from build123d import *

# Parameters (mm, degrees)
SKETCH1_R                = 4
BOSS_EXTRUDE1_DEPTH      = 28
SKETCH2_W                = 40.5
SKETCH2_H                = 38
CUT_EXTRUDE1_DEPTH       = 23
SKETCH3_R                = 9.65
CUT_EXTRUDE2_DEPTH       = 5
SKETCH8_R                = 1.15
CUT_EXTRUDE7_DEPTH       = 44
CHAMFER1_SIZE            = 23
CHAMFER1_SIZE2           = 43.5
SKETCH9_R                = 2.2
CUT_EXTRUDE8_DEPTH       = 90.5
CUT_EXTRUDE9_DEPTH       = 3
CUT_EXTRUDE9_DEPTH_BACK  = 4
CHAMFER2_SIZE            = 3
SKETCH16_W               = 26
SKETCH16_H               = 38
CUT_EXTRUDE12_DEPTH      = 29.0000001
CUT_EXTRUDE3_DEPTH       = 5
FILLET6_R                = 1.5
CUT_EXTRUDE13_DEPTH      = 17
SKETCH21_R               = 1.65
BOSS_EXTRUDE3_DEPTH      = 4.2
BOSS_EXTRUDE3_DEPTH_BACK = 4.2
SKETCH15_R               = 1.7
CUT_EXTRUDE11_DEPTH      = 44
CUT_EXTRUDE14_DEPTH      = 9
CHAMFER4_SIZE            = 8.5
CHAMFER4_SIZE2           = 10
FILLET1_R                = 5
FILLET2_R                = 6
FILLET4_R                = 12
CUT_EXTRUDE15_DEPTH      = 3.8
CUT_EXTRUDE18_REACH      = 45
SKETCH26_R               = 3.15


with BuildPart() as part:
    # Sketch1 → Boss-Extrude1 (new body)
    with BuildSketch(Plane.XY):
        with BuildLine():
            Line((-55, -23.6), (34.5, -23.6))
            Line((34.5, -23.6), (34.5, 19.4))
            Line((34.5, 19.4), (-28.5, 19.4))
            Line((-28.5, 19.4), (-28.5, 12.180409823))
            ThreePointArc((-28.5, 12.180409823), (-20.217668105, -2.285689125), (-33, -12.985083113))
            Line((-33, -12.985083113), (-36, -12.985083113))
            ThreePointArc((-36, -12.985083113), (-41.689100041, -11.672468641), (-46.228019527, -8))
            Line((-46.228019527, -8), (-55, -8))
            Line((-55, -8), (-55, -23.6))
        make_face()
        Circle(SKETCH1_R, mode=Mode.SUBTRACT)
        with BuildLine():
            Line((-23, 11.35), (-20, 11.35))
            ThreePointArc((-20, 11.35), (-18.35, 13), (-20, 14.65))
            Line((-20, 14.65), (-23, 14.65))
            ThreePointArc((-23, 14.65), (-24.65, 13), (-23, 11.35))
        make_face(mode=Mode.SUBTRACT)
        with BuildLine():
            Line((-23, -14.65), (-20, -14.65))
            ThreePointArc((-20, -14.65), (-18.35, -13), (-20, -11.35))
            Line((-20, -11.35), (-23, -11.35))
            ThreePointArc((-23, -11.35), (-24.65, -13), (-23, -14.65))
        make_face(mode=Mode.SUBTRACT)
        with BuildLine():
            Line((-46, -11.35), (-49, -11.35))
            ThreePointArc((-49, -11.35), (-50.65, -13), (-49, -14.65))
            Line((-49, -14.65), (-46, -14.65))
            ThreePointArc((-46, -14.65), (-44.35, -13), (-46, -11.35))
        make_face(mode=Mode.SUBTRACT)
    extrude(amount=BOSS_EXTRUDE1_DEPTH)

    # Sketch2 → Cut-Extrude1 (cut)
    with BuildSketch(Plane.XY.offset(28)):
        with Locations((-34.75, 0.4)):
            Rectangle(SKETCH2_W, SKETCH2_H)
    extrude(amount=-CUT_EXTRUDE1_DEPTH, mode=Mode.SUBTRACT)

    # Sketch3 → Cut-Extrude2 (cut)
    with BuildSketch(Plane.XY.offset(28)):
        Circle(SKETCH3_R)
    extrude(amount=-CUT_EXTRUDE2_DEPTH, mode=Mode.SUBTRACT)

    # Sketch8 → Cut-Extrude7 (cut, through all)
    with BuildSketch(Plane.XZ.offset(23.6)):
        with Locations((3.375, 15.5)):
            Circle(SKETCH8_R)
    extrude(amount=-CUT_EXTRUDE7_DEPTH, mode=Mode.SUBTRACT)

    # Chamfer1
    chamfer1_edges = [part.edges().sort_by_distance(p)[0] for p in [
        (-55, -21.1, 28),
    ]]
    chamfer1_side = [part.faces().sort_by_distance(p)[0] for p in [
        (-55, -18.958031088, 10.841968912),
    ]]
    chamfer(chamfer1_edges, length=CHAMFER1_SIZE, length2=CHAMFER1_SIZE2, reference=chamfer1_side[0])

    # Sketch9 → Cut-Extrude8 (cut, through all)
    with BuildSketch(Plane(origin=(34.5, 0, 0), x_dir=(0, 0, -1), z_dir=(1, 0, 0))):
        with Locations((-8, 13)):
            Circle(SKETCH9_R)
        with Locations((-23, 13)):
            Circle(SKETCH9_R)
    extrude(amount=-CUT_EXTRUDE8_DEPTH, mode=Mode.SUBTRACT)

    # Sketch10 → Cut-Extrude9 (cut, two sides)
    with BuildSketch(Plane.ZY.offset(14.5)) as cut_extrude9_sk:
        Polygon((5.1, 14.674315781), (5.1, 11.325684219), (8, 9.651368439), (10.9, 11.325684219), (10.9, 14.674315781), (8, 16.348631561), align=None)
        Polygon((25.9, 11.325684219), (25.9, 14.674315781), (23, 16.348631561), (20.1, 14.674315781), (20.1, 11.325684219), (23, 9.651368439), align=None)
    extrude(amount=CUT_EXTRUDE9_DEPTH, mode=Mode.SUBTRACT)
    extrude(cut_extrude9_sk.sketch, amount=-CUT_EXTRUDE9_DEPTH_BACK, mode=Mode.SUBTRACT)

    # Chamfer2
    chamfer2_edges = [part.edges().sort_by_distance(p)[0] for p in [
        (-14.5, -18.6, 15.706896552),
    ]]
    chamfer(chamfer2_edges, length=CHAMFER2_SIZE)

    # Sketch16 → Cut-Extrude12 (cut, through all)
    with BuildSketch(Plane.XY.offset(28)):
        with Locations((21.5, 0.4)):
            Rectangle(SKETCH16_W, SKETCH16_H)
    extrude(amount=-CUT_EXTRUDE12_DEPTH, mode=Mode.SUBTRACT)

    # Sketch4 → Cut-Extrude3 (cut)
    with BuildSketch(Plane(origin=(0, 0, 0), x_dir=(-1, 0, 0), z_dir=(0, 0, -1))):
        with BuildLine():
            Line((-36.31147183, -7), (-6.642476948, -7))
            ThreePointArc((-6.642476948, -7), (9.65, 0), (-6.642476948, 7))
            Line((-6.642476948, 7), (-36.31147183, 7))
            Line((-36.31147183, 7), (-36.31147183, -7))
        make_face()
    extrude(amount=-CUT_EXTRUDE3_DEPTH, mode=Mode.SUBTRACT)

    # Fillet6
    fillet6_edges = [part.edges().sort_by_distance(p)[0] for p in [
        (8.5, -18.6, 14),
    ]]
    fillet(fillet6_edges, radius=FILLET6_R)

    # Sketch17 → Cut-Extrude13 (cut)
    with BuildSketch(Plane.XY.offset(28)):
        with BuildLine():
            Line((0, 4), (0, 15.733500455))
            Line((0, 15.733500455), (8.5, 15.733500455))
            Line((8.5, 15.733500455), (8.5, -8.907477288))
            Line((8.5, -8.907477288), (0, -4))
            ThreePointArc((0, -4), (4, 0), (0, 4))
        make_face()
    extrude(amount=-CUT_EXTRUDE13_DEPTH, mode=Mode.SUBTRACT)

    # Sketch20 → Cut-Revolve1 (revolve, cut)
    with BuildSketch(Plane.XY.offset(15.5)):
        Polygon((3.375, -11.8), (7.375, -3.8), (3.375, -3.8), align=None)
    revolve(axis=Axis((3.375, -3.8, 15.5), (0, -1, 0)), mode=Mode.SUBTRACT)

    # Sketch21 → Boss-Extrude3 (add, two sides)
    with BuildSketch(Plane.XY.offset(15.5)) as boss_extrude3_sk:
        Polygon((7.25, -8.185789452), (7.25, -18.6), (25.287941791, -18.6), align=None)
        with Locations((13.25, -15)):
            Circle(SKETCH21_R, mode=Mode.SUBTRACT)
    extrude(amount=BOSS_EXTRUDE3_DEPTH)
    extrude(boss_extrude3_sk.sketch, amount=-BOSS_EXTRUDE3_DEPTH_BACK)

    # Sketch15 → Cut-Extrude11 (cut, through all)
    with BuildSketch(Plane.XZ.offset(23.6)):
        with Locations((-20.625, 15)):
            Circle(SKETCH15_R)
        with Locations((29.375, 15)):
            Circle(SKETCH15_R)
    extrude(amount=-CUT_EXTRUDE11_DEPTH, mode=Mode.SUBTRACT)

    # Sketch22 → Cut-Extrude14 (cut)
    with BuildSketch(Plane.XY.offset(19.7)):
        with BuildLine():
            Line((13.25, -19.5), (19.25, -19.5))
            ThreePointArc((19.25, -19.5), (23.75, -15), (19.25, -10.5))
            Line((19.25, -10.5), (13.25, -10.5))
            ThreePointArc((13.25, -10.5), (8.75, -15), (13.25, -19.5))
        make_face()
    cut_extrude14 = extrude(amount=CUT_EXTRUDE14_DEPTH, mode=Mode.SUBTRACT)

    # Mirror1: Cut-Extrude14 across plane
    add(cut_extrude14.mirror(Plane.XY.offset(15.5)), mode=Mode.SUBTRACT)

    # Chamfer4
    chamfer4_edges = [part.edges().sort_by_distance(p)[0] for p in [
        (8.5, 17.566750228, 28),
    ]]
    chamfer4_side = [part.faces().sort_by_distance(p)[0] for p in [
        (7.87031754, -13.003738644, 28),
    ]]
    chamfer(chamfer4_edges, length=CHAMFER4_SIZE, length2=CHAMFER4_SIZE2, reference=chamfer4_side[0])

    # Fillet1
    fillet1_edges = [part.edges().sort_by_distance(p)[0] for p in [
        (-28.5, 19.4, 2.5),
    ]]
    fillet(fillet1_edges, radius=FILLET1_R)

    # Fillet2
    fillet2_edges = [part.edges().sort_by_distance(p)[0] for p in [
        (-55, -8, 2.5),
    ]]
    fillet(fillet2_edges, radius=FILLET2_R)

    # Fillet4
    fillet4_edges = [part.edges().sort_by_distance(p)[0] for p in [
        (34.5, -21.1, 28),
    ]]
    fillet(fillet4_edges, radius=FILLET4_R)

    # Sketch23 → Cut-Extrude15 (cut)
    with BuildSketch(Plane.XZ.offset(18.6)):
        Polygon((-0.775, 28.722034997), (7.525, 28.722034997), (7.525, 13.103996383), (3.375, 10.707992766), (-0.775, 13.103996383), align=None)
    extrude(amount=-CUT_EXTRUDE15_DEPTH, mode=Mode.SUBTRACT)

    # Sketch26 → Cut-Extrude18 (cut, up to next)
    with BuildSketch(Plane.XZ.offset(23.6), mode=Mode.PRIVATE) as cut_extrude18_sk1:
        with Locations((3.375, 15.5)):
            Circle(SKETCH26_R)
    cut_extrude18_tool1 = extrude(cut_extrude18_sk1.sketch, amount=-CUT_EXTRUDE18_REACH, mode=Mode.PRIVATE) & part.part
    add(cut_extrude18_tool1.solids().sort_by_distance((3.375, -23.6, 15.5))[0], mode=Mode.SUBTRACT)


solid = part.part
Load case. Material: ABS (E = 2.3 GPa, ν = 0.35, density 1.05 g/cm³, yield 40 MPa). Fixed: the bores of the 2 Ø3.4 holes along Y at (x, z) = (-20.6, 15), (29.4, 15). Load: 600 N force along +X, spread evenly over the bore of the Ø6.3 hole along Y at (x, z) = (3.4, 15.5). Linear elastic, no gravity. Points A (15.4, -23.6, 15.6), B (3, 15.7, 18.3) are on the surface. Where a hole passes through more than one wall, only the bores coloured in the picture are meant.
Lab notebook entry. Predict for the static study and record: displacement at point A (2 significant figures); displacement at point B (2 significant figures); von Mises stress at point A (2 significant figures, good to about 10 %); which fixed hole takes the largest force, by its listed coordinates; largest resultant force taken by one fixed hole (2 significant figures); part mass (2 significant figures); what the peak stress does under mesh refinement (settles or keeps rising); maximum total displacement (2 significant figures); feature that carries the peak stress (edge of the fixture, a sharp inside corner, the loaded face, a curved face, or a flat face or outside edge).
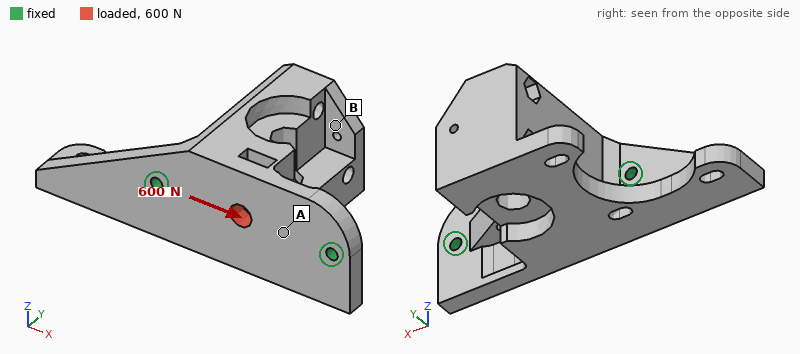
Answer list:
25 µm
13 µm
4.3 MPa
(-20.6, 15)
330 N
31 g
keeps rising
45 µm
edge of the fixture
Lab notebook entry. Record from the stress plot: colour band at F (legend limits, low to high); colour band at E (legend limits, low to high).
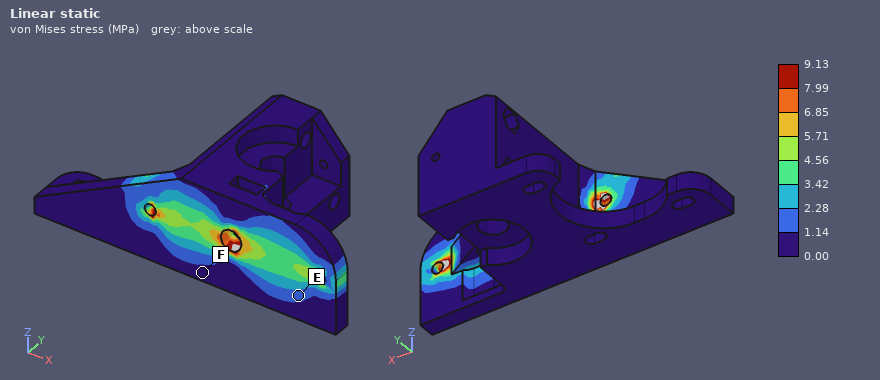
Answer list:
0.00 to 1.14 MPa
1.14 to 2.28 MPa
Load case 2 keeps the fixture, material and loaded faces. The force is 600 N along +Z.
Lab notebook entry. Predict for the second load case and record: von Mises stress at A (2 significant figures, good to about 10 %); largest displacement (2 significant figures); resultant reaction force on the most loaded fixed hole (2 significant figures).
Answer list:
4.5 MPa
0.13 mm
310 N
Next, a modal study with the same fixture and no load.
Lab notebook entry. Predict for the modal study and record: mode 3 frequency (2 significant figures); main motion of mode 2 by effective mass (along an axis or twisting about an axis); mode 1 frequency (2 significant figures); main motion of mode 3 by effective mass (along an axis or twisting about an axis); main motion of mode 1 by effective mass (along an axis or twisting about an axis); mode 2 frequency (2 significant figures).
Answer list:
1800 Hz
along X
570 Hz
along Y
along Z
1400 Hz
